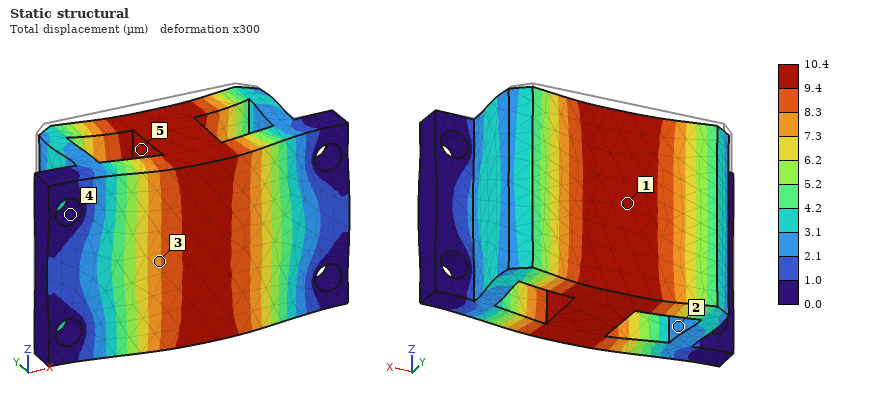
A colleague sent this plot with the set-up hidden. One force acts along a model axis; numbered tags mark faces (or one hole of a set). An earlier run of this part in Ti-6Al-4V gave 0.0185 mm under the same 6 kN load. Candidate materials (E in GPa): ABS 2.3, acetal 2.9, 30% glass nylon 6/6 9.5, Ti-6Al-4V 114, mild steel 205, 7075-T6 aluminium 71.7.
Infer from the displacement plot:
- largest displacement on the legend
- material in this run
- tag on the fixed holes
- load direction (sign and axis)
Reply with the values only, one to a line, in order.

10.4 µm
mild steel
4
-Y
